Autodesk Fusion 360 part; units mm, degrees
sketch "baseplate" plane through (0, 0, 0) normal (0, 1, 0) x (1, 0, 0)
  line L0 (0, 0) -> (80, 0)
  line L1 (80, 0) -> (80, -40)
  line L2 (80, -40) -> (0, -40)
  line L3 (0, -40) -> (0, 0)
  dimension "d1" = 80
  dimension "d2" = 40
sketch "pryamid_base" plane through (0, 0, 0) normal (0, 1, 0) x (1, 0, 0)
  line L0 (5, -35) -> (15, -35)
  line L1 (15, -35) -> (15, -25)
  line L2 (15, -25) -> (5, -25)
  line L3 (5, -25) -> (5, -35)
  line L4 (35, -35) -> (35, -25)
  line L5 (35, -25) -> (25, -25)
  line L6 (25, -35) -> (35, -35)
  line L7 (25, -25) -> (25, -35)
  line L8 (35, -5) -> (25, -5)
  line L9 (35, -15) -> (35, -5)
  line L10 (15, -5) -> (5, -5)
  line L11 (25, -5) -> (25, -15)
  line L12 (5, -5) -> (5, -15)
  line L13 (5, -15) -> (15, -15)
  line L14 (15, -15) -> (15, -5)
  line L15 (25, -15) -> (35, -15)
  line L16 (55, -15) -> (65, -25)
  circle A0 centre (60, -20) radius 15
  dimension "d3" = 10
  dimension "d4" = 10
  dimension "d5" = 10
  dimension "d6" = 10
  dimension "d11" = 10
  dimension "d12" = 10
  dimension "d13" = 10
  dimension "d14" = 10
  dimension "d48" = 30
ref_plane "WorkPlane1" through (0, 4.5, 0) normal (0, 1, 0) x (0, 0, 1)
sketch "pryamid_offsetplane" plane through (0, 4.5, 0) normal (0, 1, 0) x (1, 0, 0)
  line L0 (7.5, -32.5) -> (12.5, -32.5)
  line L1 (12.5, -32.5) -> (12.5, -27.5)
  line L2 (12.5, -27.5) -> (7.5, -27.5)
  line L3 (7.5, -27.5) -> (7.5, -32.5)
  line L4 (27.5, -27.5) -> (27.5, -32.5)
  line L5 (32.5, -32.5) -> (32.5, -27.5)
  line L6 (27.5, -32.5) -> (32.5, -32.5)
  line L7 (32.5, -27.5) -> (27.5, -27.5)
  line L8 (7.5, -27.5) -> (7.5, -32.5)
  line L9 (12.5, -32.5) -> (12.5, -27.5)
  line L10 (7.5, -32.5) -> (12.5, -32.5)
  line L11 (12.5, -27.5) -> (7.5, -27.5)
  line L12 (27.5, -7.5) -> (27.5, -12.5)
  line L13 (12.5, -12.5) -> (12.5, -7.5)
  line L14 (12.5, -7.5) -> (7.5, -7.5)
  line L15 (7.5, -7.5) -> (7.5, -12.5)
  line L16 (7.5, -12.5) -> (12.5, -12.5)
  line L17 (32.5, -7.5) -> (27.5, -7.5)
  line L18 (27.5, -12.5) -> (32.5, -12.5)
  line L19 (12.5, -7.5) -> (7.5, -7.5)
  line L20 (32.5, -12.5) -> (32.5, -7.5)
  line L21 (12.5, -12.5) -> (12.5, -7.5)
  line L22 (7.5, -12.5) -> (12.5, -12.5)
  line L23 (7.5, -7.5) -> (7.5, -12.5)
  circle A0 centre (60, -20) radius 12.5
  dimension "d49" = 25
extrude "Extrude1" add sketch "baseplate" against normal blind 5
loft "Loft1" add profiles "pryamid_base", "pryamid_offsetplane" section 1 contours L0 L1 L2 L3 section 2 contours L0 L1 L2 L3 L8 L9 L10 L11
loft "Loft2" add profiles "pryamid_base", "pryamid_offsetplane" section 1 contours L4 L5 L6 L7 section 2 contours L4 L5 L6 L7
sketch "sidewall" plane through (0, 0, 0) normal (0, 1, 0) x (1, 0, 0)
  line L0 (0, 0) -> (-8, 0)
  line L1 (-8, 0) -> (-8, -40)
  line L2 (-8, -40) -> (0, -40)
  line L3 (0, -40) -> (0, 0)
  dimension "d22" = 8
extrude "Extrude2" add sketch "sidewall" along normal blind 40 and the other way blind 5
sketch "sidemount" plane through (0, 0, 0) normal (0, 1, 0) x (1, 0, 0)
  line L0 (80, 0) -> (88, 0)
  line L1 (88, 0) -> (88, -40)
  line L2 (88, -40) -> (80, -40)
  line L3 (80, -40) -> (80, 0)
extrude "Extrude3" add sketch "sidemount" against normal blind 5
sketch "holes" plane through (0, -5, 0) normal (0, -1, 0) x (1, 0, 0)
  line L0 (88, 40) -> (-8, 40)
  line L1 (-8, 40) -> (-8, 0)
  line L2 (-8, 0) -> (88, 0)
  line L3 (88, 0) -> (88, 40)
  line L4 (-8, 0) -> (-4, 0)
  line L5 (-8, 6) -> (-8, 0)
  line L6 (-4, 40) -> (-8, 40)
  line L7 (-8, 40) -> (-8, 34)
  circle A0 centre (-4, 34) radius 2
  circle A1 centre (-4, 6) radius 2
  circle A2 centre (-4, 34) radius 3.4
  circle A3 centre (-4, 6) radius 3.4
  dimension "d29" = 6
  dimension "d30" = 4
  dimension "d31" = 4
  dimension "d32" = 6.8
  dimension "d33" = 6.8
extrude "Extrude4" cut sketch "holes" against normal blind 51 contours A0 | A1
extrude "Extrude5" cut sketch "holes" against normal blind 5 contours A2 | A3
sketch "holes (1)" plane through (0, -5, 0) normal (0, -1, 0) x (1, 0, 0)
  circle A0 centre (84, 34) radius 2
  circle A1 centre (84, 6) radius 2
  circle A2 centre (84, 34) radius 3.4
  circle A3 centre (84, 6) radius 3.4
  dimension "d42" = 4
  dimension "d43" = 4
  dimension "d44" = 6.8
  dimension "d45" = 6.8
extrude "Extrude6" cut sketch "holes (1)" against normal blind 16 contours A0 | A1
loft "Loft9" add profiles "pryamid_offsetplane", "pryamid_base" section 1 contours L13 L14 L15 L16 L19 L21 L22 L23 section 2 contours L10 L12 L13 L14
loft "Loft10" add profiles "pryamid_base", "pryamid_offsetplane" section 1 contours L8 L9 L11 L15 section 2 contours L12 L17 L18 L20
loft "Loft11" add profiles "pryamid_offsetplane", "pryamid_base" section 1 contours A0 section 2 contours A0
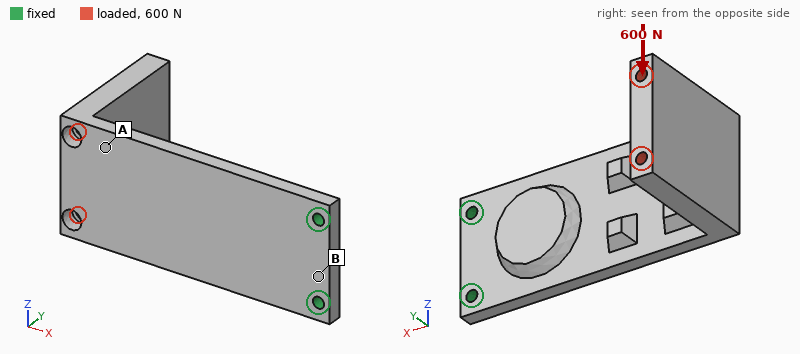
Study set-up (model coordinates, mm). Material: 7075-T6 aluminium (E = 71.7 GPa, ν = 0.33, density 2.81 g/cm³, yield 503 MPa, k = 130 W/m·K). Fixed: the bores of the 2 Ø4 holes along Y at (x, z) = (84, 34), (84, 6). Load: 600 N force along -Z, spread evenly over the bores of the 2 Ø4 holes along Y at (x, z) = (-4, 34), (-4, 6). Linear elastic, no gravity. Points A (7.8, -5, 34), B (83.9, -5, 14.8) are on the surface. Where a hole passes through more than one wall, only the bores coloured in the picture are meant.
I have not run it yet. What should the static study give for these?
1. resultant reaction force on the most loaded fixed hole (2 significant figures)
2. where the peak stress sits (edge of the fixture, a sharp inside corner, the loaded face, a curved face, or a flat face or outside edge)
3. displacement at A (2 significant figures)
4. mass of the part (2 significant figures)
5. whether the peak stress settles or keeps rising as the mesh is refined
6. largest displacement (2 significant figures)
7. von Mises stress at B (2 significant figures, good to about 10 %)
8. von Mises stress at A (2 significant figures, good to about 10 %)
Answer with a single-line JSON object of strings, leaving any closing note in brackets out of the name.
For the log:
{"resultant reaction force on the most loaded fixed hole": "1.9 kN", "where the peak stress sits": "edge of the fixture", "displacement at A": "0.17 mm", "mass of the part": "96 g", "whether the peak stress settles or keeps rising as the mesh is refined": "keeps rising", "largest displacement": "0.71 mm", "von Mises stress at B": "14 MPa", "von Mises stress at A": "42 MPa"}
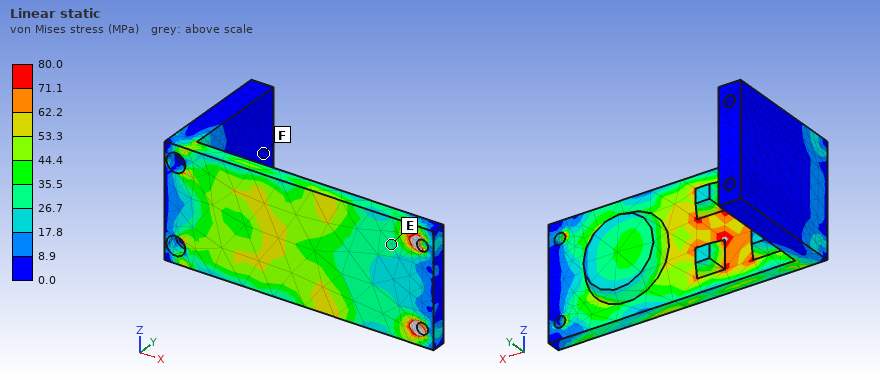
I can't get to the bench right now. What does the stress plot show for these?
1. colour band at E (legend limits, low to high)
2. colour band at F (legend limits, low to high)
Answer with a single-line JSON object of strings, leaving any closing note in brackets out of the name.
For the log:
{"colour band at E": "26.7 to 35.5 MPa", "colour band at F": "0.0 to 8.9 MPa"}
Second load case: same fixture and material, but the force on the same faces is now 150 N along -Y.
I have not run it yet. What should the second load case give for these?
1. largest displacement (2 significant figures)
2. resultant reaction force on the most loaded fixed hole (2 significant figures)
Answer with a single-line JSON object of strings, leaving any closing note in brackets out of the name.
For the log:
{"largest displacement": "1.0 mm", "resultant reaction force on the most loaded fixed hole": "110 N"}
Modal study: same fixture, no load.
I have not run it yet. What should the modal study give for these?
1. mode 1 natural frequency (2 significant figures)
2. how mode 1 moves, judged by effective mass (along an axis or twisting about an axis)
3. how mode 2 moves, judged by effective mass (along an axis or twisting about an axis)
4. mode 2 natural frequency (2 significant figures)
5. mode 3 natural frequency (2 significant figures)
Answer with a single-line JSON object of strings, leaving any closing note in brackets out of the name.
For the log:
{"mode 1 natural frequency": "300 Hz", "how mode 1 moves, judged by effective mass": "along Y", "how mode 2 moves, judged by effective mass": "along Z", "mode 2 natural frequency": "900 Hz", "mode 3 natural frequency": "1200 Hz"}
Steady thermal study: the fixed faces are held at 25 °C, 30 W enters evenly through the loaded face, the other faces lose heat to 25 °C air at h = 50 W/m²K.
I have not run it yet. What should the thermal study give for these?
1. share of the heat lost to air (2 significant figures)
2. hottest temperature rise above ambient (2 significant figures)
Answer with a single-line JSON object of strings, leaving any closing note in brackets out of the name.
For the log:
{"share of the heat lost to air": "64 %", "hottest temperature rise above ambient": "53 K"}
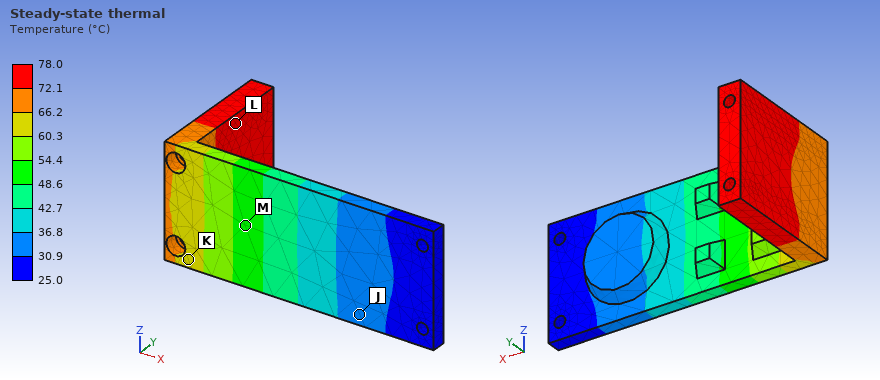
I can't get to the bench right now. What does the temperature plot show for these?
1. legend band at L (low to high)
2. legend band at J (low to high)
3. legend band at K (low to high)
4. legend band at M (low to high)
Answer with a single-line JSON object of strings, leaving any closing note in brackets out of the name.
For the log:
{"legend band at L": "72.1 to 78.0 °C", "legend band at J": "30.9 to 36.8 °C", "legend band at K": "60.3 to 66.2 °C", "legend band at M": "48.6 to 54.4 °C"}
